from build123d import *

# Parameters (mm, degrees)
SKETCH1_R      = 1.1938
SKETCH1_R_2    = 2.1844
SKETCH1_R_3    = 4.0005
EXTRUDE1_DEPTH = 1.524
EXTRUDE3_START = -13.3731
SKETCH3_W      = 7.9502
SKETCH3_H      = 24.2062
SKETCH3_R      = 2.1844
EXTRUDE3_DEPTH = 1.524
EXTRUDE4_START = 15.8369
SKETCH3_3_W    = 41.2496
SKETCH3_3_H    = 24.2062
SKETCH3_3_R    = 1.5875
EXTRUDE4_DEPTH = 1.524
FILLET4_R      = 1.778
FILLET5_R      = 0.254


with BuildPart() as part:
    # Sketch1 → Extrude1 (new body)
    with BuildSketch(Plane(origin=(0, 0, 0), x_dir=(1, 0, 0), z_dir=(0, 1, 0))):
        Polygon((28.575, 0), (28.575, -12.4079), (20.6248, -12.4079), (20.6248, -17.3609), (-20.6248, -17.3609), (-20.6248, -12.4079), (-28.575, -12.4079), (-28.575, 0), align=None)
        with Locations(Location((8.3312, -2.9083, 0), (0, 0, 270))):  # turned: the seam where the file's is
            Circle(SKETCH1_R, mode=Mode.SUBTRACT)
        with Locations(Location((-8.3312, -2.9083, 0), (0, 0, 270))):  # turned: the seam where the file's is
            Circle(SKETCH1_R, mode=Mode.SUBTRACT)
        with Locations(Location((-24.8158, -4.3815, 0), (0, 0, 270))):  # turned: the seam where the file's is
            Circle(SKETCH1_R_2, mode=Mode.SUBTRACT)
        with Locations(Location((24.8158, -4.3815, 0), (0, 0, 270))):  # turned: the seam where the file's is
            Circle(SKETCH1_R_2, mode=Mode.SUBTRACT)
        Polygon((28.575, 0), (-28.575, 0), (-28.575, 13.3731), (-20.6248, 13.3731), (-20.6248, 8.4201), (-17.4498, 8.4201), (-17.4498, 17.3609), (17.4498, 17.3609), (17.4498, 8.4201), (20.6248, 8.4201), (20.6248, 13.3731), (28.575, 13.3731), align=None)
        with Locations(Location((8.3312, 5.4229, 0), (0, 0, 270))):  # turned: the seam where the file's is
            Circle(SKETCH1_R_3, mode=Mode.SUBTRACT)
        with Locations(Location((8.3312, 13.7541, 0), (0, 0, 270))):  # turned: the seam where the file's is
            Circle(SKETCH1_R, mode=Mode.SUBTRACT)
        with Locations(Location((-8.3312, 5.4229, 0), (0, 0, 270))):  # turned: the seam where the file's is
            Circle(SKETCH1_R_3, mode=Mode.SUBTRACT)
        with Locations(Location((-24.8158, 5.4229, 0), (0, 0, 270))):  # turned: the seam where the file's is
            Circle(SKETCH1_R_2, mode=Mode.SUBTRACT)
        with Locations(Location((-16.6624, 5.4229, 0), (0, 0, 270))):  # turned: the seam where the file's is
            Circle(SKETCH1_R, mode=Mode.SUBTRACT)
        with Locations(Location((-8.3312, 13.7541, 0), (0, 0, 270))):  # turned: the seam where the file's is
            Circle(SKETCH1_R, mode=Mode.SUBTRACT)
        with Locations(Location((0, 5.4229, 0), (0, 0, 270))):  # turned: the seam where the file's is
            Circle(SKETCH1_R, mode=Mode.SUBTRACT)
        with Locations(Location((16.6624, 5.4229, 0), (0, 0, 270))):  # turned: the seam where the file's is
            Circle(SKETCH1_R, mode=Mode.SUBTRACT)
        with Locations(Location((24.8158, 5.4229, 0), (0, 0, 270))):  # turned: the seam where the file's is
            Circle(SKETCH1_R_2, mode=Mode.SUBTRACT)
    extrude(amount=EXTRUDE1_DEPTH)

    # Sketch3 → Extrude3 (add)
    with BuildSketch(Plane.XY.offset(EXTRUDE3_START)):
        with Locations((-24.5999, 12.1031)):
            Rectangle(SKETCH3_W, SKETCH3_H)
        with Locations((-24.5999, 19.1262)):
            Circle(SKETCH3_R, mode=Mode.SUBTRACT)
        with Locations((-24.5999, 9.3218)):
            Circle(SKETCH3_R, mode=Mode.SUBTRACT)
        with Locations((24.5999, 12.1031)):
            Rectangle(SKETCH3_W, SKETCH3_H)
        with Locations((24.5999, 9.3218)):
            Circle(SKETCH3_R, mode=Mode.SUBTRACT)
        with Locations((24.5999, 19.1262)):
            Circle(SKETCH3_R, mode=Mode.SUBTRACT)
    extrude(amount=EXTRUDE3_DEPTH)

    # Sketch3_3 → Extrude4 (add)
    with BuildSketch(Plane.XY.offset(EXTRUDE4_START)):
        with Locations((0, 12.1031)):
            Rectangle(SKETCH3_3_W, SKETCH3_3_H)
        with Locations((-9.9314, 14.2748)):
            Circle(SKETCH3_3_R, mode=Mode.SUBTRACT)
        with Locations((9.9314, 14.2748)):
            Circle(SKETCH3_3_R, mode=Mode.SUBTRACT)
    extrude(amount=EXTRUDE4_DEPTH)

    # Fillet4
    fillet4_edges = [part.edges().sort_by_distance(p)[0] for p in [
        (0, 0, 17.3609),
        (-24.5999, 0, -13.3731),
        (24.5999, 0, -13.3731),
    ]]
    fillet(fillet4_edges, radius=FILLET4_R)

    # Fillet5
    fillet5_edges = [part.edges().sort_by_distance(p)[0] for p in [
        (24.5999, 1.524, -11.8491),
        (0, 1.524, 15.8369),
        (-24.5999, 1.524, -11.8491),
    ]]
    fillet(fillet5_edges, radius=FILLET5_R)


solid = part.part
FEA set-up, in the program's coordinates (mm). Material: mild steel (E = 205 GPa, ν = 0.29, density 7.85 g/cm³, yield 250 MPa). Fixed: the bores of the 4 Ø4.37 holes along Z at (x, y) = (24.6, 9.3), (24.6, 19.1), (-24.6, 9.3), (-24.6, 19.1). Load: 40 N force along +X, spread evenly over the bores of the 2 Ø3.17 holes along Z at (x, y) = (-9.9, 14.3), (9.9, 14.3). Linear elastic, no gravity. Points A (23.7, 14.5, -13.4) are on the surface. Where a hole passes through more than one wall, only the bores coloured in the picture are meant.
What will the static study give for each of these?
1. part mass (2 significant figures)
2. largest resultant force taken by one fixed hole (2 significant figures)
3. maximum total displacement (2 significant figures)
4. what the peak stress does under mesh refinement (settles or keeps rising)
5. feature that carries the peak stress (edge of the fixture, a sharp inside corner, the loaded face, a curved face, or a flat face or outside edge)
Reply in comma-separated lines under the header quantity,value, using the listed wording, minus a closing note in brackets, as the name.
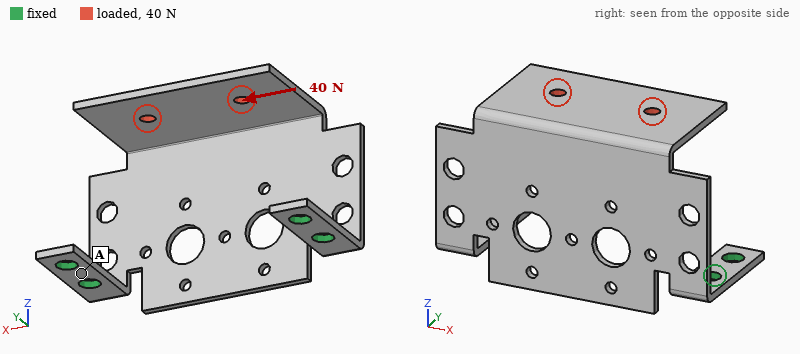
quantity,value
part mass,33 g
largest resultant force taken by one fixed hole,33 N
maximum total displacement,93 µm
what the peak stress does under mesh refinement,keeps rising
feature that carries the peak stress,edge of the fixture
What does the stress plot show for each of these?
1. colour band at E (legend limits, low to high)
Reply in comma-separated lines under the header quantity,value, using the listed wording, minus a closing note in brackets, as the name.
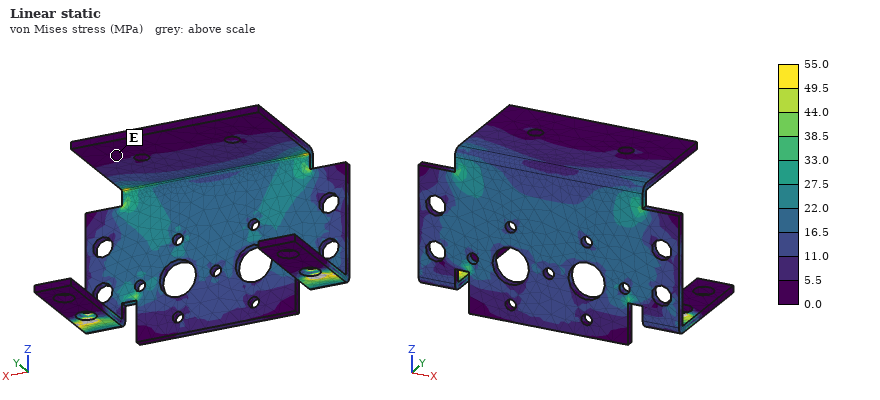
quantity,value
colour band at E,0.0 to 5.5 MPa
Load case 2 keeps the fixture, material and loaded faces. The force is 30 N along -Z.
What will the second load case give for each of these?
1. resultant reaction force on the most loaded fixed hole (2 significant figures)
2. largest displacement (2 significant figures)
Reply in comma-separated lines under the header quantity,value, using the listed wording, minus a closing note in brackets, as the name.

quantity,value
resultant reaction force on the most loaded fixed hole,16 N
largest displacement,0.31 mm
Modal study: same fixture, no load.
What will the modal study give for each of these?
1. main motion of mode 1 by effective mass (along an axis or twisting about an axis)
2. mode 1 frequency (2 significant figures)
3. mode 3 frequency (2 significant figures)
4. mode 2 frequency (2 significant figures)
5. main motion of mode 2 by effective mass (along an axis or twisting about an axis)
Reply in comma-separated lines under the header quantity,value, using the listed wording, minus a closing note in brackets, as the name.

quantity,value
main motion of mode 1 by effective mass,along Y
mode 1 frequency,310 Hz
mode 3 frequency,1300 Hz
mode 2 frequency,1000 Hz
main motion of mode 2 by effective mass,along X
